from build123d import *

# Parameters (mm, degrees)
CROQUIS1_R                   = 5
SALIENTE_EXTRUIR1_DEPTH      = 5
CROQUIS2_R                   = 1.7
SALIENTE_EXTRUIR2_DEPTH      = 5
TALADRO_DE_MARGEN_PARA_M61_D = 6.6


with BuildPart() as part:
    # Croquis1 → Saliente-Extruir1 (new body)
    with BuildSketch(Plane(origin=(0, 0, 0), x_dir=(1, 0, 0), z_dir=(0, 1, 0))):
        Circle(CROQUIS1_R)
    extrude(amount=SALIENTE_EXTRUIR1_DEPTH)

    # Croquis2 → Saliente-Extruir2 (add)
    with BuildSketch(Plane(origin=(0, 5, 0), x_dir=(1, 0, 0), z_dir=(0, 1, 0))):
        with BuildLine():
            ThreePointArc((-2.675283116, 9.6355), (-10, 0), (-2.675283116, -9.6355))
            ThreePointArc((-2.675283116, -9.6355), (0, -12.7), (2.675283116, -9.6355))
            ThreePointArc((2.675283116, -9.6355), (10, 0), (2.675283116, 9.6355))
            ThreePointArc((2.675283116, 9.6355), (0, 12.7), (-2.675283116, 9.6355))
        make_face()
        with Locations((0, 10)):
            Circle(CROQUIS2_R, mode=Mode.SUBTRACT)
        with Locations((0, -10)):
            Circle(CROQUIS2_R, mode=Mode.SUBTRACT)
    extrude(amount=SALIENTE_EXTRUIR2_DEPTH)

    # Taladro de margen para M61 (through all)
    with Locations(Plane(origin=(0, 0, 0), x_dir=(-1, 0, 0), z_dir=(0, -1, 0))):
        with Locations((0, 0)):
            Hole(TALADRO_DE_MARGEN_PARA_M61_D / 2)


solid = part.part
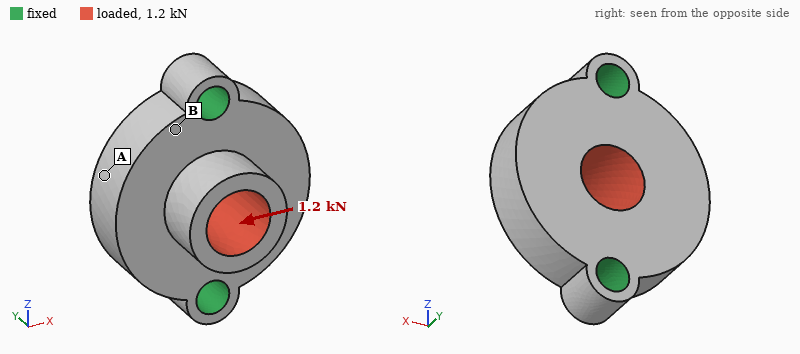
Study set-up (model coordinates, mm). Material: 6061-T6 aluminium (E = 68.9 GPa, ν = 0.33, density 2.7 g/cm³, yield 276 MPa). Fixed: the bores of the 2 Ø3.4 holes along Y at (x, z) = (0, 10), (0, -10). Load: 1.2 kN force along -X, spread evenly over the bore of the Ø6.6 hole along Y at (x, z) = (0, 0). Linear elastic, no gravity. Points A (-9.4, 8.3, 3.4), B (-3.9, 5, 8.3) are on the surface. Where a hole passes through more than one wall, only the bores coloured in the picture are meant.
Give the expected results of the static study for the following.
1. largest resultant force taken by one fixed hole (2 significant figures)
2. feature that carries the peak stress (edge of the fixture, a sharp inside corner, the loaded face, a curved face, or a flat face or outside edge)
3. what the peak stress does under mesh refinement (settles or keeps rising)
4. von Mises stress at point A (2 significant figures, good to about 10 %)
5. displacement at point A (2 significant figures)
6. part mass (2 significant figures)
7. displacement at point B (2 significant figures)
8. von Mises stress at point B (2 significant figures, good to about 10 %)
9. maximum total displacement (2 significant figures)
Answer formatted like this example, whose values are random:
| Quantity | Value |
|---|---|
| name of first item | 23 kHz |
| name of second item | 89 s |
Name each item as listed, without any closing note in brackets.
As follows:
| Quantity | Value |
|---|---|
| largest resultant force taken by one fixed hole | 600 N |
| feature that carries the peak stress | edge of the fixture |
| what the peak stress does under mesh refinement | keeps rising |
| von Mises stress at point A | 12 MPa |
| displacement at point A | 8.2 µm |
| part mass | 4.5 g |
| displacement at point B | 3.0 µm |
| von Mises stress at point B | 35 MPa |
| maximum total displacement | 15 µm |
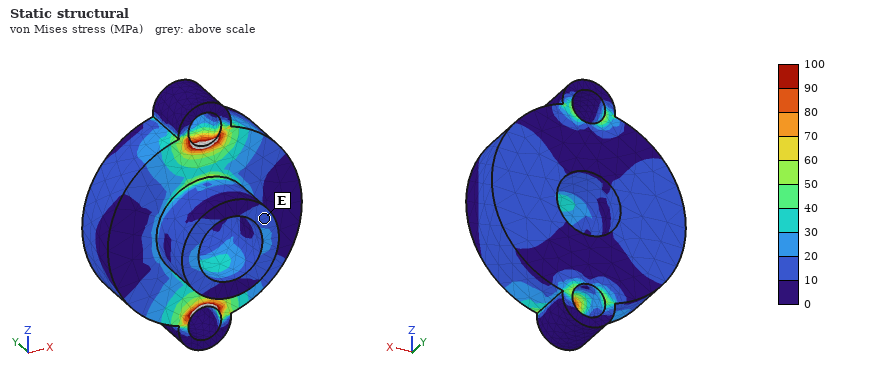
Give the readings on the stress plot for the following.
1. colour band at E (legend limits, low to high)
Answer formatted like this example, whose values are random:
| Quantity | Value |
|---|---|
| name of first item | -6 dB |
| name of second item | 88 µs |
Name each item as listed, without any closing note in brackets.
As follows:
| Quantity | Value |
|---|---|
| colour band at E | 10 to 20 MPa |
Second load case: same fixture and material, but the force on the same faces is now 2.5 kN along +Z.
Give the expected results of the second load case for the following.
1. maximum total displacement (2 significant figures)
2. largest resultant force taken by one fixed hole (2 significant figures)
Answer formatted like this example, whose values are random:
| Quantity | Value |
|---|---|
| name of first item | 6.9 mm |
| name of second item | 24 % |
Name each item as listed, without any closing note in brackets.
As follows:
| Quantity | Value |
|---|---|
| maximum total displacement | 14 µm |
| largest resultant force taken by one fixed hole | 1.3 kN |
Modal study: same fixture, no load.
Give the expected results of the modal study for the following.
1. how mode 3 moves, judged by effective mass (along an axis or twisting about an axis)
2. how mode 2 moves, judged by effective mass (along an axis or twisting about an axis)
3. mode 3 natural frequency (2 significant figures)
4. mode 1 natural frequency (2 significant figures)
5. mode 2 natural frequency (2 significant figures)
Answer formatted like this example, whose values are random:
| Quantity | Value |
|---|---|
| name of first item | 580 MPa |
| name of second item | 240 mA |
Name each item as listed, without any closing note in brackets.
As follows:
| Quantity | Value |
|---|---|
| how mode 3 moves, judged by effective mass | along X |
| how mode 2 moves, judged by effective mass | along Y |
| mode 3 natural frequency | 59 kHz |
| mode 1 natural frequency | 26 kHz |
| mode 2 natural frequency | 35 kHz |
